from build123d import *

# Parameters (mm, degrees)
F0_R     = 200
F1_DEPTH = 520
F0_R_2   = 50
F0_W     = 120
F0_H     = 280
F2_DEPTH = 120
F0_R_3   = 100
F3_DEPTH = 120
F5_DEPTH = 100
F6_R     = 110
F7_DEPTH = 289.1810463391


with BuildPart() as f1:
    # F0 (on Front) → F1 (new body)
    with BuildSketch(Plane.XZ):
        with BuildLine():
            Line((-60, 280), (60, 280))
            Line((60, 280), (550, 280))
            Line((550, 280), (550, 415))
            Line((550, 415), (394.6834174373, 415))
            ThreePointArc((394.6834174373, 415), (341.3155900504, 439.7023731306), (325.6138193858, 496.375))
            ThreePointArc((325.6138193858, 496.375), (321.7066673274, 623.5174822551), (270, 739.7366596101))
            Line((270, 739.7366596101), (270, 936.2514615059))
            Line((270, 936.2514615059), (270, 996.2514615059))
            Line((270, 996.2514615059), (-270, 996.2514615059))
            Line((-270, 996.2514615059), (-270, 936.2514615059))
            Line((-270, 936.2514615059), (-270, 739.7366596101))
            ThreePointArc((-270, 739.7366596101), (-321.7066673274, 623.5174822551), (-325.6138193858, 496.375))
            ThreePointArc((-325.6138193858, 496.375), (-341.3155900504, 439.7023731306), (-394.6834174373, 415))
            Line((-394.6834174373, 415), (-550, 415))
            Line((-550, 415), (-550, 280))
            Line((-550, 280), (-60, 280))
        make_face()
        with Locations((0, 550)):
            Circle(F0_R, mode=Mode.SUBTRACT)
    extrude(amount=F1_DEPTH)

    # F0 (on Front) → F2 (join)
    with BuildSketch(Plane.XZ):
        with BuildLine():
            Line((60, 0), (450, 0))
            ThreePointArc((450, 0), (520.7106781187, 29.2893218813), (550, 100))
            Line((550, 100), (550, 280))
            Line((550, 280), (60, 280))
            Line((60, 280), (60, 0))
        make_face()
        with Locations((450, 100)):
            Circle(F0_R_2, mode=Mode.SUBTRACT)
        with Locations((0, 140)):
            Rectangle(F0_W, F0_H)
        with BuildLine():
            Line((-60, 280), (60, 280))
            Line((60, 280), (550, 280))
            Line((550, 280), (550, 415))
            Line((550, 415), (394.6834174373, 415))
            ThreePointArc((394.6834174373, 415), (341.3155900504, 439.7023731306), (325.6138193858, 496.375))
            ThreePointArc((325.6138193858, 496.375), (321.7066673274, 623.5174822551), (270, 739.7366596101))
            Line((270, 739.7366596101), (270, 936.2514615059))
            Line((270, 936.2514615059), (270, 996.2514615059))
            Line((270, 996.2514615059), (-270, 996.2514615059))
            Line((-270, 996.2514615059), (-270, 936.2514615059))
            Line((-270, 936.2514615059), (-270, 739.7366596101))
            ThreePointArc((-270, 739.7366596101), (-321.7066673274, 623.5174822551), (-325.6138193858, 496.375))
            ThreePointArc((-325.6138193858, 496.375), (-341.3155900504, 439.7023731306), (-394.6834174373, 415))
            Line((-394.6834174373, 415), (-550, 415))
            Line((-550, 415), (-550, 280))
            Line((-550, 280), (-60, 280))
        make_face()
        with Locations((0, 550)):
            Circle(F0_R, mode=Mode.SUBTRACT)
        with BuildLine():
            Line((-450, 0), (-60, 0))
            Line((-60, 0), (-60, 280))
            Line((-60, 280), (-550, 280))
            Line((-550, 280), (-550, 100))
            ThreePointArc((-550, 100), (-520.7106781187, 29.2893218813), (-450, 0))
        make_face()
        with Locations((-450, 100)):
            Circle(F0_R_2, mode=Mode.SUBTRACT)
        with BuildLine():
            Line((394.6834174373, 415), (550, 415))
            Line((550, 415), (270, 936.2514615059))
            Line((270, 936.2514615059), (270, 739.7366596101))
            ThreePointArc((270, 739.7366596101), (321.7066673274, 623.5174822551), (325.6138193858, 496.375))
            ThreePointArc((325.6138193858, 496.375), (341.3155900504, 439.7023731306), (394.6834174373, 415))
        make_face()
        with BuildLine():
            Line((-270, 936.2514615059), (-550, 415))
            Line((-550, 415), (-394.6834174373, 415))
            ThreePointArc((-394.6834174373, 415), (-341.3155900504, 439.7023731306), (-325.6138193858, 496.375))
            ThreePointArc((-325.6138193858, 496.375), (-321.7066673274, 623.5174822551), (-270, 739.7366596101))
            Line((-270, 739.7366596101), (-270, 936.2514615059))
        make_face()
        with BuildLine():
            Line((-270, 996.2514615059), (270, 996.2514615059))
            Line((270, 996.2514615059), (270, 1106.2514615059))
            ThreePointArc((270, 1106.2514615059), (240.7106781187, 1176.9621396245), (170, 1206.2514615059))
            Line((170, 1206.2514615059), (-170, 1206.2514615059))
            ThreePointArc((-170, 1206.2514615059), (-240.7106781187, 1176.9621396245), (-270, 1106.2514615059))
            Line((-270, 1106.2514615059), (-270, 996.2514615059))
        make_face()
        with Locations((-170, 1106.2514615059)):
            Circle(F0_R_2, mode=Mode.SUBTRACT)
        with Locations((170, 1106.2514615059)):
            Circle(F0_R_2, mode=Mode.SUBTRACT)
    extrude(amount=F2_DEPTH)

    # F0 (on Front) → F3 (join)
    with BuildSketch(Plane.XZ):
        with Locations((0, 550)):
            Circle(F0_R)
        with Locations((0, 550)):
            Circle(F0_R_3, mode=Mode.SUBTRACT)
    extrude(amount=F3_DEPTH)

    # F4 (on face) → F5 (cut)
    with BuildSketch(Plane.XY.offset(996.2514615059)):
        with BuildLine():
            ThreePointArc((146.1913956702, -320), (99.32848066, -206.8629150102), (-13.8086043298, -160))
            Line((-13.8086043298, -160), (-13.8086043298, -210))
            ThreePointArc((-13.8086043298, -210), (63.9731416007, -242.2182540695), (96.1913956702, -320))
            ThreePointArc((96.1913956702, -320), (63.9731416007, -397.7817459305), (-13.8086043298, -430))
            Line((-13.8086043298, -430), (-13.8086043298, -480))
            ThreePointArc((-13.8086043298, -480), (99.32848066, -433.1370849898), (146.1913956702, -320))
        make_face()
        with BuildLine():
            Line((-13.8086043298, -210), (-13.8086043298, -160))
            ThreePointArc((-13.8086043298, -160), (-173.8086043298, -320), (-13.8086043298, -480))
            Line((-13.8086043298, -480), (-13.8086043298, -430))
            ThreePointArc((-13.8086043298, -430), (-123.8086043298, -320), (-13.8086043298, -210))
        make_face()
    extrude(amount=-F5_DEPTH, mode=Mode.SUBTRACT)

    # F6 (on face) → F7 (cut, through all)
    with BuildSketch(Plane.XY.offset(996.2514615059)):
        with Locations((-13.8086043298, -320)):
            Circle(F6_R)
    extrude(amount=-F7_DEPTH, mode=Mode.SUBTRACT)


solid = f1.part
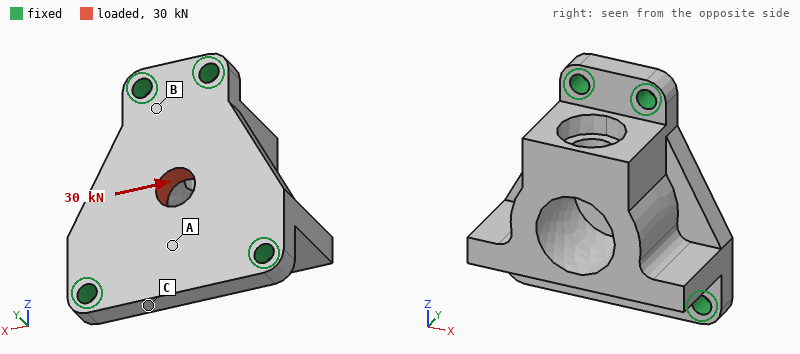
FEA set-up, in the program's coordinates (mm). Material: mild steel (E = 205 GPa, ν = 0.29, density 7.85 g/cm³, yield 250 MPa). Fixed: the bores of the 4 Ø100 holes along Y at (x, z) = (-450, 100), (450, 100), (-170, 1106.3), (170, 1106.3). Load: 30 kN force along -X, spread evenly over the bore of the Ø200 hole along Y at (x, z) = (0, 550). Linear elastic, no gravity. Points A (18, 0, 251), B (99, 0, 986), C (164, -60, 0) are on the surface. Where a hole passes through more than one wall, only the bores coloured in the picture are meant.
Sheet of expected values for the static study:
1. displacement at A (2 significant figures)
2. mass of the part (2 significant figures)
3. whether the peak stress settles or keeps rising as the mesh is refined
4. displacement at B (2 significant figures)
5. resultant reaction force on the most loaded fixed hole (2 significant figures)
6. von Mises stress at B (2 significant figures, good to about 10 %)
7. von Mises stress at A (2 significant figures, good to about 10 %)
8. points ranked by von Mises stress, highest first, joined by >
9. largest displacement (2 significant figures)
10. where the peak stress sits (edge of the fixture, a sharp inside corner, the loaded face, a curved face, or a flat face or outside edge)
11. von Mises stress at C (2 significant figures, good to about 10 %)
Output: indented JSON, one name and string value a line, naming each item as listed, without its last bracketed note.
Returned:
{
  "displacement at A": "0.51 µm",
  "mass of the part": "2000 kg",
  "whether the peak stress settles or keeps rising as the mesh is refined": "keeps rising",
  "displacement at B": "0.25 µm",
  "resultant reaction force on the most loaded fixed hole": "10 kN",
  "von Mises stress at B": "0.37 MPa",
  "von Mises stress at A": "0.25 MPa",
  "points ranked by von Mises stress, highest first, joined by >": "B > A > C",
  "largest displacement": "1.2 µm",
  "where the peak stress sits": "edge of the fixture",
  "von Mises stress at C": "0.12 MPa"
}
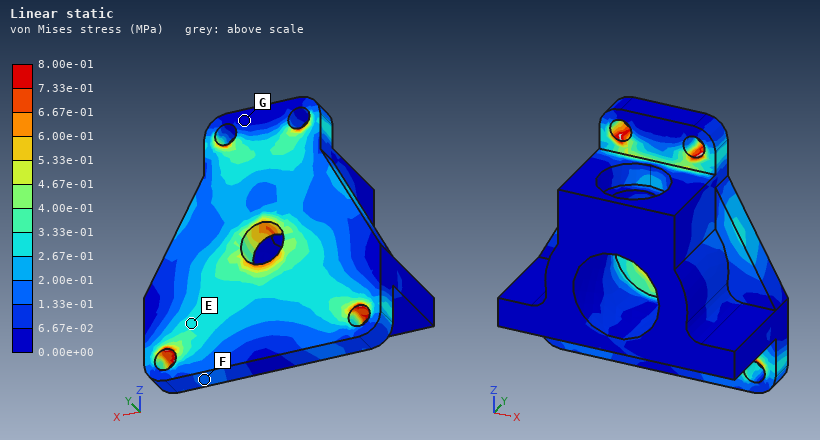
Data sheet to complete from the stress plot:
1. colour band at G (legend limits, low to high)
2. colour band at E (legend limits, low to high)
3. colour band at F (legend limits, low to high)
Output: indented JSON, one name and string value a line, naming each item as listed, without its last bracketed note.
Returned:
{
  "colour band at G": "0.00e+00 to 6.67e-02 MPa",
  "colour band at E": "2.67e-01 to 3.33e-01 MPa",
  "colour band at F": "1.33e-01 to 2.00e-01 MPa"
}
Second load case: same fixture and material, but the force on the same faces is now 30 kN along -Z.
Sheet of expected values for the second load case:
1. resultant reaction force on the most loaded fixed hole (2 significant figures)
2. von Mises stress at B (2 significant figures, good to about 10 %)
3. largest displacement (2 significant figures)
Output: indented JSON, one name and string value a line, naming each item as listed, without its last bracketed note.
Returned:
{
  "resultant reaction force on the most loaded fixed hole": "8.2 kN",
  "von Mises stress at B": "0.23 MPa",
  "largest displacement": "0.94 µm"
}
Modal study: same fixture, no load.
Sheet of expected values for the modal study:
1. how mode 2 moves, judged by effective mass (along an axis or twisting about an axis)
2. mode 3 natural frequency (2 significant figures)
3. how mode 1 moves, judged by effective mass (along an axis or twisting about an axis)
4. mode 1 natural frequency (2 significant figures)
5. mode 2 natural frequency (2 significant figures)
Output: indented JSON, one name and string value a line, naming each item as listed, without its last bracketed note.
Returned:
{
  "how mode 2 moves, judged by effective mass": "along Y",
  "mode 3 natural frequency": "780 Hz",
  "how mode 1 moves, judged by effective mass": "along X",
  "mode 1 natural frequency": "490 Hz",
  "mode 2 natural frequency": "530 Hz"
}
